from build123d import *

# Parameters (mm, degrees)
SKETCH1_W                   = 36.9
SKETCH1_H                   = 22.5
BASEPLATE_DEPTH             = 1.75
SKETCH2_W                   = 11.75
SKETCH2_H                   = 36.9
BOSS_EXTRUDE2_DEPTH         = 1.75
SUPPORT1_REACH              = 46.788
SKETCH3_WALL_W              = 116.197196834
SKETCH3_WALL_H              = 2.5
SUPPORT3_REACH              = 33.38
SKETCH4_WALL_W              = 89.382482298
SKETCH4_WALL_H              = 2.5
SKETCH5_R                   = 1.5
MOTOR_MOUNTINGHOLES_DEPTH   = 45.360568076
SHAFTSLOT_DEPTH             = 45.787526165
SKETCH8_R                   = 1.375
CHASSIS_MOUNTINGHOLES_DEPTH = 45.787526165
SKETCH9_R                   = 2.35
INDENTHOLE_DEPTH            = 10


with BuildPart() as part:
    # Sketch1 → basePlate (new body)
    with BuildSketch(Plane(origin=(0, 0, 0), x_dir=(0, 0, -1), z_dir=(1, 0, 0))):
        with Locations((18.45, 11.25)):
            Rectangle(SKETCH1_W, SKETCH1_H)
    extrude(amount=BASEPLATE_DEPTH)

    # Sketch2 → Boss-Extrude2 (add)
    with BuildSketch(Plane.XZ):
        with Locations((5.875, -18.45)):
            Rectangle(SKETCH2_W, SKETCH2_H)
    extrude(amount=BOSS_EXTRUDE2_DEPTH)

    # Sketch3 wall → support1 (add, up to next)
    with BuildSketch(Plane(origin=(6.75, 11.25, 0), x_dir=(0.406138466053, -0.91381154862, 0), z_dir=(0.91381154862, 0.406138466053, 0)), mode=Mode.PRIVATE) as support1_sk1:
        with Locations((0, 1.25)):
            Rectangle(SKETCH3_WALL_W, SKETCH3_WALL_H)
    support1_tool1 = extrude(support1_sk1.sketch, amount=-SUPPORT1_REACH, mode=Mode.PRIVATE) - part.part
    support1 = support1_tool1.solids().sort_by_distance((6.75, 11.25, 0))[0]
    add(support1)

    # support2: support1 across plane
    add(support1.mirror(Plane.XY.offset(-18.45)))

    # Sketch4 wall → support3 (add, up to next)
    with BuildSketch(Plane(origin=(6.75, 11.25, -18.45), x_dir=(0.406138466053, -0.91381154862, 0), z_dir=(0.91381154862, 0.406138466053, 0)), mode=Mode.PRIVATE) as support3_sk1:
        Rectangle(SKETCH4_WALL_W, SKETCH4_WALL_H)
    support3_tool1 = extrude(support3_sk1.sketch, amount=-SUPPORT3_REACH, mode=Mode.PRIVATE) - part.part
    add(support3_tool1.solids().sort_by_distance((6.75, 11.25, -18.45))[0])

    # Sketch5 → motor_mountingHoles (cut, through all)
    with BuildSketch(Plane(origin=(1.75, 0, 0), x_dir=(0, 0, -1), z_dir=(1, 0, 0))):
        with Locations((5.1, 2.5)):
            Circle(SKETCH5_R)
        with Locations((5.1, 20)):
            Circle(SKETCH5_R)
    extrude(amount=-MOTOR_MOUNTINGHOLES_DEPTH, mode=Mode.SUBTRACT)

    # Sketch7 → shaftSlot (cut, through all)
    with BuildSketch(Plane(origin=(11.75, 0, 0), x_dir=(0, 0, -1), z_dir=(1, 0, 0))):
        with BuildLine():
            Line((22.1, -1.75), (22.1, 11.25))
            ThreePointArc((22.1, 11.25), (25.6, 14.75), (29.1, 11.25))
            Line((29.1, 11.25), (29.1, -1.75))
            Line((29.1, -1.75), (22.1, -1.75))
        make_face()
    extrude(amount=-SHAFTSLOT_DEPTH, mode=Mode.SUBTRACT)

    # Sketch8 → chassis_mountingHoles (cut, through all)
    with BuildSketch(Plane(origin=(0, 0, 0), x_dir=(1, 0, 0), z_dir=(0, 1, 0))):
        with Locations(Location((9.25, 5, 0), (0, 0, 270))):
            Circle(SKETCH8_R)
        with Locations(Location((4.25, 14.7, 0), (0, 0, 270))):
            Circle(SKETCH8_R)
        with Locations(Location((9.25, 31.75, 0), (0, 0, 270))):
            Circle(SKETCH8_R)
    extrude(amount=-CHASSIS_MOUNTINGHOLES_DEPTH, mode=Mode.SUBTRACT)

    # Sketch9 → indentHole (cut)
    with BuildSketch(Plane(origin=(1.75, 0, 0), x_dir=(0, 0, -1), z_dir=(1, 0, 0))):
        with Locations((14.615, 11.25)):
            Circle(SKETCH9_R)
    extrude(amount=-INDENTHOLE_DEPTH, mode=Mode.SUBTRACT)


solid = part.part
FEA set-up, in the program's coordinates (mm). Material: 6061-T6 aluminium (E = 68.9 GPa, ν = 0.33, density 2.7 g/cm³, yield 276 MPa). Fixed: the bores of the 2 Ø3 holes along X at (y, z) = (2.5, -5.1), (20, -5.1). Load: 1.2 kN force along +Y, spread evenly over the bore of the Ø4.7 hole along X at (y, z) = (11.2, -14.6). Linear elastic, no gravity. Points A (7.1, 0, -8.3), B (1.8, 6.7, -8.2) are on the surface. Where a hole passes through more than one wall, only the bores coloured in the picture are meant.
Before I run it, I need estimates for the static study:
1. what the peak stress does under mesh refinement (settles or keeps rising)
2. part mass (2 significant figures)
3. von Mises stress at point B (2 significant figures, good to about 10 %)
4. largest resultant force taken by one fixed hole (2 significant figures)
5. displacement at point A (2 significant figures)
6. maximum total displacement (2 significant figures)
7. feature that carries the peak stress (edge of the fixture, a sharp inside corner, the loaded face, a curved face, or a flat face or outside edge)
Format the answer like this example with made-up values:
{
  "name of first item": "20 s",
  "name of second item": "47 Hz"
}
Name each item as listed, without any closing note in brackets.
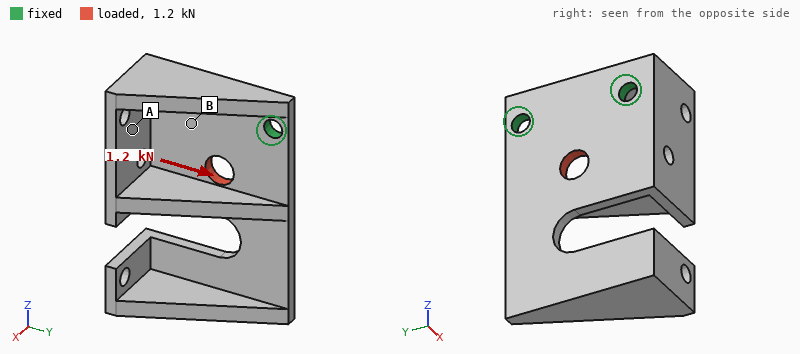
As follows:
{
  "what the peak stress does under mesh refinement": "keeps rising",
  "part mass": "7.2 g",
  "von Mises stress at point B": "56 MPa",
  "largest resultant force taken by one fixed hole": "870 N",
  "displacement at point A": "6.6 µm",
  "maximum total displacement": "32 µm",
  "feature that carries the peak stress": "edge of the fixture"
}
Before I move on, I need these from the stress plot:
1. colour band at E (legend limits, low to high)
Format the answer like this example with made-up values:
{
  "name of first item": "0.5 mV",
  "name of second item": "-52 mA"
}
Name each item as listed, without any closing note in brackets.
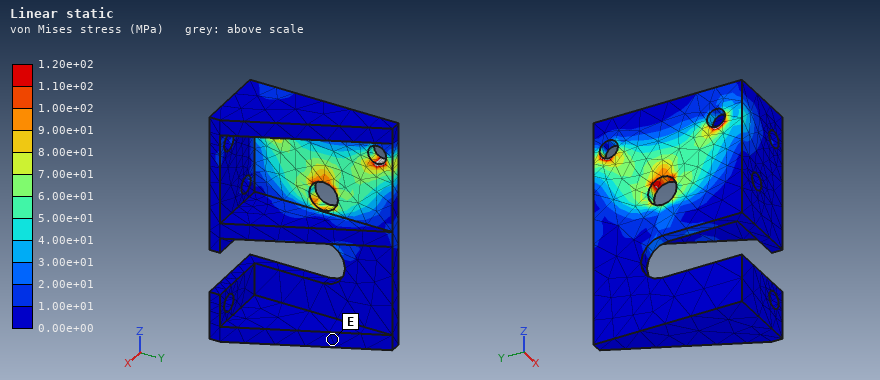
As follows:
{
  "colour band at E": "0.00e+00 to 1.00e+01 MPa"
}
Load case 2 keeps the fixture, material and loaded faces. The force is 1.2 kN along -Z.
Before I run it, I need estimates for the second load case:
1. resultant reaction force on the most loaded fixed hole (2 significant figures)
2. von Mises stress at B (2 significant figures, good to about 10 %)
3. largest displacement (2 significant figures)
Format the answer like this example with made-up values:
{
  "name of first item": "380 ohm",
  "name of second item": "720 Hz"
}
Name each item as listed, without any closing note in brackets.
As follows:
{
  "resultant reaction force on the most loaded fixed hole": "620 N",
  "von Mises stress at B": "42 MPa",
  "largest displacement": "19 µm"
}
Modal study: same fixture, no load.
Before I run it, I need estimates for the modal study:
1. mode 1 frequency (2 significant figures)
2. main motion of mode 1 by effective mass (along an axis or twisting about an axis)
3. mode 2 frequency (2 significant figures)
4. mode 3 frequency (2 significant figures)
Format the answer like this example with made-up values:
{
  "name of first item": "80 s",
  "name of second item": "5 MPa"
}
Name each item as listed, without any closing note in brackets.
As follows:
{
  "mode 1 frequency": "980 Hz",
  "main motion of mode 1 by effective mass": "along X",
  "mode 2 frequency": "2200 Hz",
  "mode 3 frequency": "3800 Hz"
}
